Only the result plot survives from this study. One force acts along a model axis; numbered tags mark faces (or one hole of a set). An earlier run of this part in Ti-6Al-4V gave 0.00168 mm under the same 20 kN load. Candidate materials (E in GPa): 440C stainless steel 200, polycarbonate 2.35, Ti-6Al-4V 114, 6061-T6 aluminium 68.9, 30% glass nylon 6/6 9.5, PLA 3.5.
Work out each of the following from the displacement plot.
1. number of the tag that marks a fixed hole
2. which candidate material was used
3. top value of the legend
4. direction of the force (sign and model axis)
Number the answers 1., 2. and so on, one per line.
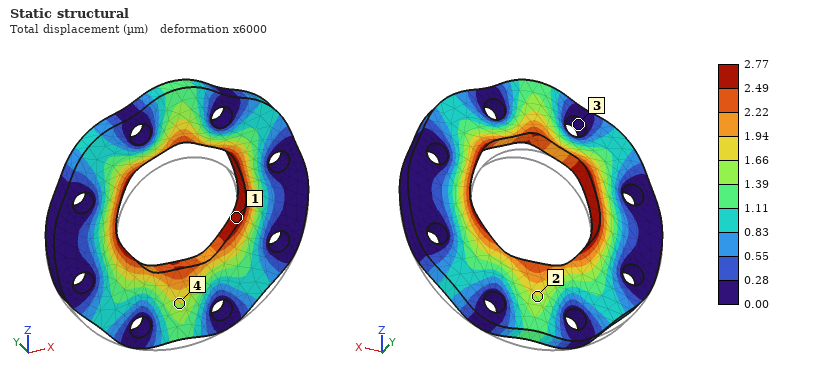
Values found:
1. 3
2. 6061-T6 aluminium
3. 2.77 µm
4. +Z
